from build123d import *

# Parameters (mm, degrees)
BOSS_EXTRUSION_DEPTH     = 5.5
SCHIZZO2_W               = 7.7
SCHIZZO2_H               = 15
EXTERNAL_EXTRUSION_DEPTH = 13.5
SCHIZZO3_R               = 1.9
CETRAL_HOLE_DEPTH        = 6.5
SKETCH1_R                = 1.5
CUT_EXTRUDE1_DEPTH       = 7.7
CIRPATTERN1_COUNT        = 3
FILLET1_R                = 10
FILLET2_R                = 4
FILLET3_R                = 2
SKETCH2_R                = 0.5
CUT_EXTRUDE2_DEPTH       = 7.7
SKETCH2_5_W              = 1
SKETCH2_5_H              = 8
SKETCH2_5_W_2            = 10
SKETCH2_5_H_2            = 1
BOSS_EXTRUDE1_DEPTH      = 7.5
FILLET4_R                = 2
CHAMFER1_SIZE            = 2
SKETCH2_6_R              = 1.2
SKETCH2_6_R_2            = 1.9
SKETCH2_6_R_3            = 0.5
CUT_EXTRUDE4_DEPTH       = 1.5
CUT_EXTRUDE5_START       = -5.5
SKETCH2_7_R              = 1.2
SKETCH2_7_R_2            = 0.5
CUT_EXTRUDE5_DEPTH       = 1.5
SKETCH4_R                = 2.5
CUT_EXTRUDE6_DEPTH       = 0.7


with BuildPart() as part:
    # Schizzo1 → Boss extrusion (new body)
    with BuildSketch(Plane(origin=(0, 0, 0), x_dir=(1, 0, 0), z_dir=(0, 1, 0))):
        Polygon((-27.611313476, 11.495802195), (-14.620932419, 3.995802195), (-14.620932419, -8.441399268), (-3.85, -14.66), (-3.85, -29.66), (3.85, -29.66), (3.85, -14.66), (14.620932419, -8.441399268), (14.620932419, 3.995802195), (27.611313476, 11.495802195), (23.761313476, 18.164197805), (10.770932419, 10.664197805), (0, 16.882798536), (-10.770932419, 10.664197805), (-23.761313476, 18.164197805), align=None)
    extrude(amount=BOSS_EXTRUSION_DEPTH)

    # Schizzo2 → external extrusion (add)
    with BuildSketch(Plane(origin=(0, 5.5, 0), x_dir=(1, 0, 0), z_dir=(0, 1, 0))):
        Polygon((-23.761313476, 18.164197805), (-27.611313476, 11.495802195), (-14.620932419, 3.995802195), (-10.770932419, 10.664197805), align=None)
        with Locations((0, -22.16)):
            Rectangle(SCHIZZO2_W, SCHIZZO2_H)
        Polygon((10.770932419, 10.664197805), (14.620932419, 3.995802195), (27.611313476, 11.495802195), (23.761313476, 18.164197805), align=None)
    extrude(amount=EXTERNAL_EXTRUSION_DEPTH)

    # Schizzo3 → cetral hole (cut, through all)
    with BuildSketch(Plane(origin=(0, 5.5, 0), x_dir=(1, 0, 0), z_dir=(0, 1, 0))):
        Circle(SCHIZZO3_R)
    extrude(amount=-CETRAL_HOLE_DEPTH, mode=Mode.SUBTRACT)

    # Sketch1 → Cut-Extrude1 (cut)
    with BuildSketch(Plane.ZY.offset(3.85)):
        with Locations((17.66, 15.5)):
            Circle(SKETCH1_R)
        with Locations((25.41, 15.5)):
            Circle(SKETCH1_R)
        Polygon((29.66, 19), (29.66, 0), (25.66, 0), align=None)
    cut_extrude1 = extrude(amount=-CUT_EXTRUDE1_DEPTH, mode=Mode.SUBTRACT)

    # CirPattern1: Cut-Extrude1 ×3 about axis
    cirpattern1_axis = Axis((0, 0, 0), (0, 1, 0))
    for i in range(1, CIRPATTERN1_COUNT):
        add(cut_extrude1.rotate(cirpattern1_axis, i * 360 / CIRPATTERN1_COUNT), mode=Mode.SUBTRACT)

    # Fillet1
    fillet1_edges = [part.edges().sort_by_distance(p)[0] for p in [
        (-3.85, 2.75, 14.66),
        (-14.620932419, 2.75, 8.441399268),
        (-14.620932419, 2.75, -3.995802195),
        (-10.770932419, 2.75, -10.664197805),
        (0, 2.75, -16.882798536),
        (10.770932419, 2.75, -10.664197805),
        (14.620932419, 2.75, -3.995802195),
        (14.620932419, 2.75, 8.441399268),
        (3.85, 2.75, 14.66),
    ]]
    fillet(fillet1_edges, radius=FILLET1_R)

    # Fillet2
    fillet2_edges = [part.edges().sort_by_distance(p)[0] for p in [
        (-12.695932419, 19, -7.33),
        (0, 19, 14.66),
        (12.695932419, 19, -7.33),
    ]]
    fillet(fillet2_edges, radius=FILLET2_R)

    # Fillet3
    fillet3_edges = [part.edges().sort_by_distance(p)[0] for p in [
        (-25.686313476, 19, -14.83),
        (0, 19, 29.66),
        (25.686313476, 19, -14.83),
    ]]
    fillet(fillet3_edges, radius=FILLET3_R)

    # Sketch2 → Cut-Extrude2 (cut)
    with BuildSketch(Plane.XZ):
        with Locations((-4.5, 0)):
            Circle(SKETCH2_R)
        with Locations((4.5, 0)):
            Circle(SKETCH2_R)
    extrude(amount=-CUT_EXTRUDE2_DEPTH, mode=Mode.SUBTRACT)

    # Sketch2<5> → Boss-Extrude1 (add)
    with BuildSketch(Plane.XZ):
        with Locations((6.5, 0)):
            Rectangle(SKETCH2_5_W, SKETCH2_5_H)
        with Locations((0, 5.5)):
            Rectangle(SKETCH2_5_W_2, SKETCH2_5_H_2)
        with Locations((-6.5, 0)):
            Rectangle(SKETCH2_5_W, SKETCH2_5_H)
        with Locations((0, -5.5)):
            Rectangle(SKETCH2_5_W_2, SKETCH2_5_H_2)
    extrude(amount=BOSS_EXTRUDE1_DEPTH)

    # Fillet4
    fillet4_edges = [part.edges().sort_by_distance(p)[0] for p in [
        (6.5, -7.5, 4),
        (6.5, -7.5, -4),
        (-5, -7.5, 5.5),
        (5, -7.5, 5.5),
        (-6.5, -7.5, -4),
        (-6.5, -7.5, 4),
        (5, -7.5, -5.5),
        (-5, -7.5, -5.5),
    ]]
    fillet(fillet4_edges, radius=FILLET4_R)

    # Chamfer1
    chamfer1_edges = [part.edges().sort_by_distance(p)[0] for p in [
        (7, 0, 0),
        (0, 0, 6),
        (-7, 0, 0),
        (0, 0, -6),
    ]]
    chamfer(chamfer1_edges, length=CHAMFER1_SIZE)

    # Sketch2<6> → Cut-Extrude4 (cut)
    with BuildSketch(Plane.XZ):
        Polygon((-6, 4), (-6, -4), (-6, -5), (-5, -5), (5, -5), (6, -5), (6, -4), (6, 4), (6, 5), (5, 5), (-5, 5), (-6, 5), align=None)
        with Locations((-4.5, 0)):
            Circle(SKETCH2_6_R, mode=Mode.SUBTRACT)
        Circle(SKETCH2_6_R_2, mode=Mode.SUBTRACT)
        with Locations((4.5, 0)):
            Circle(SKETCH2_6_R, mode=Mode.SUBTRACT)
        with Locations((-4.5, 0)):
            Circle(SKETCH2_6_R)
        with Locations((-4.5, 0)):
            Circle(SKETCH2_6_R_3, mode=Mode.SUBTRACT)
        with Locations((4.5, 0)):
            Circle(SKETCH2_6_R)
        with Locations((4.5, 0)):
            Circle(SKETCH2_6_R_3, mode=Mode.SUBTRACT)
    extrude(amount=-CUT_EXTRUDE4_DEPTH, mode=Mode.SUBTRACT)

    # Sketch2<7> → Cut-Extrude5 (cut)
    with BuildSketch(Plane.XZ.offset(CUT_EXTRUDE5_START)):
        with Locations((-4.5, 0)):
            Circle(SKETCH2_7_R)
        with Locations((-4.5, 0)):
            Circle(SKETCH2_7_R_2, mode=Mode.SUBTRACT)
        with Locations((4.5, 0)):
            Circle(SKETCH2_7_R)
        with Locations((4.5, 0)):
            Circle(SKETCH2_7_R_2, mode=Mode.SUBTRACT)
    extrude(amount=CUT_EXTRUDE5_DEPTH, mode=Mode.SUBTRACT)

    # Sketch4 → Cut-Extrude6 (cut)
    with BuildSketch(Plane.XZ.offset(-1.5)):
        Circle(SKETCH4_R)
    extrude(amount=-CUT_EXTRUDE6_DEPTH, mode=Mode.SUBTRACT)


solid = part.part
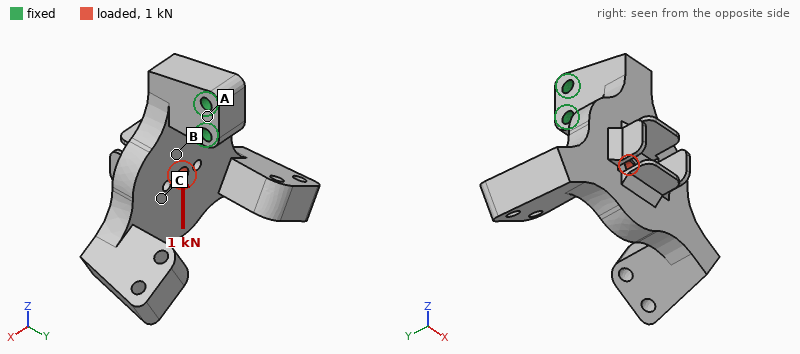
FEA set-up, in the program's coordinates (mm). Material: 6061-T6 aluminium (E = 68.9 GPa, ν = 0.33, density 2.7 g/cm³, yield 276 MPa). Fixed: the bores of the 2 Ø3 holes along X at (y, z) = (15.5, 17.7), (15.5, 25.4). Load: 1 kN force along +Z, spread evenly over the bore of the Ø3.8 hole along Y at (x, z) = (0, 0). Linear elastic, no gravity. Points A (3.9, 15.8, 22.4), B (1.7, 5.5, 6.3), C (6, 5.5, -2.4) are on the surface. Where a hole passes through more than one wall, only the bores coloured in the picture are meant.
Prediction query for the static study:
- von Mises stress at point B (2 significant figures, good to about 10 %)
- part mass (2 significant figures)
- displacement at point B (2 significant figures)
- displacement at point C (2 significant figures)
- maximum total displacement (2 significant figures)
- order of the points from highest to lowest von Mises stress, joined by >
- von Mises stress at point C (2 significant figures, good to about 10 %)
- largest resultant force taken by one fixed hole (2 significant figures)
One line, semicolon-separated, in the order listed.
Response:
26 MPa; 25 g; 14 µm; 15 µm; 18 µm; B > C > A; 9.9 MPa; 1.3 kN
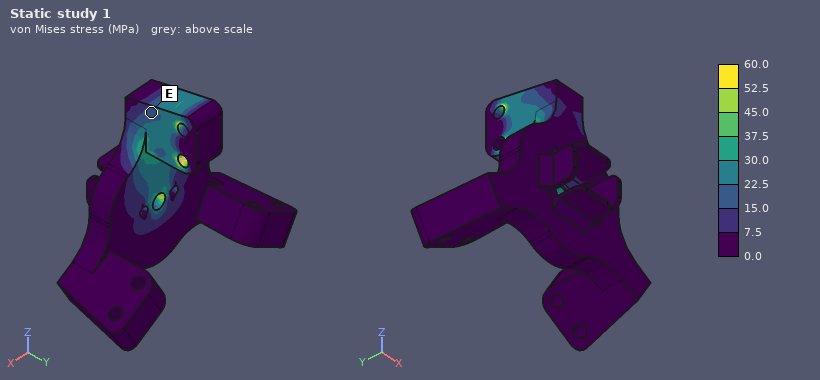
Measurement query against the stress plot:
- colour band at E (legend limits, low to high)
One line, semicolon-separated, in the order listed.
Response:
15.0 to 22.5 MPa
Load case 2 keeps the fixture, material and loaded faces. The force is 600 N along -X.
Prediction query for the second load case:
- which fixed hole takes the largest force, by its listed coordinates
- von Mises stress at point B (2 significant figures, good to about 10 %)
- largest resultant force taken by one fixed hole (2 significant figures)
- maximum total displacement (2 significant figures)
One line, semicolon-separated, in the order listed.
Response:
(15.5, 17.7); 25 MPa; 1.3 kN; 0.29 mm
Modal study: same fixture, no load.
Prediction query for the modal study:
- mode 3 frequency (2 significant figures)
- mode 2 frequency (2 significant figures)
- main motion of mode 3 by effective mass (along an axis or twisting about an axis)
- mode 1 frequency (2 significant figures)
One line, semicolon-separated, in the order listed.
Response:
2000 Hz; 1600 Hz; twisting about Z; 1500 Hz
